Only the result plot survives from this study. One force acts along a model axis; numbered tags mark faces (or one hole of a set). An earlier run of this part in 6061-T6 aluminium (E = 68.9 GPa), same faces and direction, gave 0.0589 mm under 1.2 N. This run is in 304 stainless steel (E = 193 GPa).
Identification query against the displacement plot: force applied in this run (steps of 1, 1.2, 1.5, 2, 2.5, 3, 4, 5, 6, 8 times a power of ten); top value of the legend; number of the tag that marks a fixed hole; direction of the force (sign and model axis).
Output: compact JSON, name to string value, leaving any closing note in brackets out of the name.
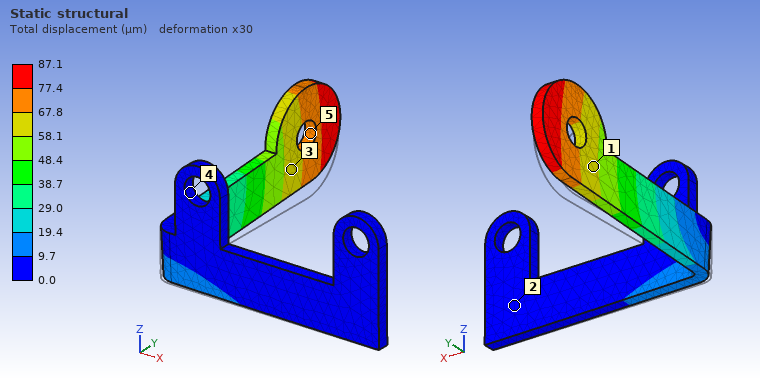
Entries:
{"force applied in this run": "5 N", "top value of the legend": "87.1 µm", "number of the tag that marks a fixed hole": "4", "direction of the force": "+Z"}
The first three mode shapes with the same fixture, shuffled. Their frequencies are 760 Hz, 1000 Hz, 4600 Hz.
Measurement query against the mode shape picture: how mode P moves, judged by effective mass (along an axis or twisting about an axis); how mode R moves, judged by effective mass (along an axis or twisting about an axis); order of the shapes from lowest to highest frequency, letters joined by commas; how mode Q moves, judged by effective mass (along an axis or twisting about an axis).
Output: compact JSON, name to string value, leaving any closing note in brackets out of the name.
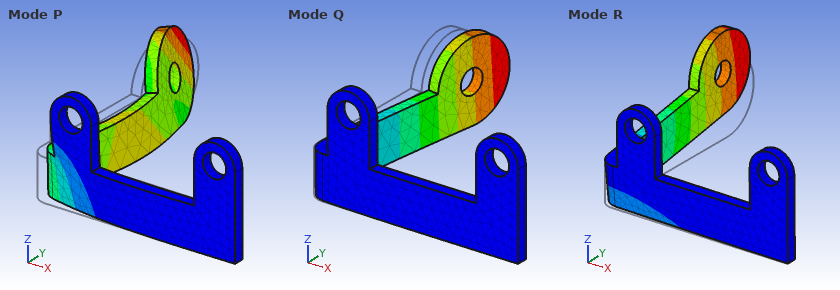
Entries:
{"how mode P moves, judged by effective mass": "along Y", "how mode R moves, judged by effective mass": "along Z", "order of the shapes from lowest to highest frequency, letters joined by commas": "Q, R, P", "how mode Q moves, judged by effective mass": "along X"}
